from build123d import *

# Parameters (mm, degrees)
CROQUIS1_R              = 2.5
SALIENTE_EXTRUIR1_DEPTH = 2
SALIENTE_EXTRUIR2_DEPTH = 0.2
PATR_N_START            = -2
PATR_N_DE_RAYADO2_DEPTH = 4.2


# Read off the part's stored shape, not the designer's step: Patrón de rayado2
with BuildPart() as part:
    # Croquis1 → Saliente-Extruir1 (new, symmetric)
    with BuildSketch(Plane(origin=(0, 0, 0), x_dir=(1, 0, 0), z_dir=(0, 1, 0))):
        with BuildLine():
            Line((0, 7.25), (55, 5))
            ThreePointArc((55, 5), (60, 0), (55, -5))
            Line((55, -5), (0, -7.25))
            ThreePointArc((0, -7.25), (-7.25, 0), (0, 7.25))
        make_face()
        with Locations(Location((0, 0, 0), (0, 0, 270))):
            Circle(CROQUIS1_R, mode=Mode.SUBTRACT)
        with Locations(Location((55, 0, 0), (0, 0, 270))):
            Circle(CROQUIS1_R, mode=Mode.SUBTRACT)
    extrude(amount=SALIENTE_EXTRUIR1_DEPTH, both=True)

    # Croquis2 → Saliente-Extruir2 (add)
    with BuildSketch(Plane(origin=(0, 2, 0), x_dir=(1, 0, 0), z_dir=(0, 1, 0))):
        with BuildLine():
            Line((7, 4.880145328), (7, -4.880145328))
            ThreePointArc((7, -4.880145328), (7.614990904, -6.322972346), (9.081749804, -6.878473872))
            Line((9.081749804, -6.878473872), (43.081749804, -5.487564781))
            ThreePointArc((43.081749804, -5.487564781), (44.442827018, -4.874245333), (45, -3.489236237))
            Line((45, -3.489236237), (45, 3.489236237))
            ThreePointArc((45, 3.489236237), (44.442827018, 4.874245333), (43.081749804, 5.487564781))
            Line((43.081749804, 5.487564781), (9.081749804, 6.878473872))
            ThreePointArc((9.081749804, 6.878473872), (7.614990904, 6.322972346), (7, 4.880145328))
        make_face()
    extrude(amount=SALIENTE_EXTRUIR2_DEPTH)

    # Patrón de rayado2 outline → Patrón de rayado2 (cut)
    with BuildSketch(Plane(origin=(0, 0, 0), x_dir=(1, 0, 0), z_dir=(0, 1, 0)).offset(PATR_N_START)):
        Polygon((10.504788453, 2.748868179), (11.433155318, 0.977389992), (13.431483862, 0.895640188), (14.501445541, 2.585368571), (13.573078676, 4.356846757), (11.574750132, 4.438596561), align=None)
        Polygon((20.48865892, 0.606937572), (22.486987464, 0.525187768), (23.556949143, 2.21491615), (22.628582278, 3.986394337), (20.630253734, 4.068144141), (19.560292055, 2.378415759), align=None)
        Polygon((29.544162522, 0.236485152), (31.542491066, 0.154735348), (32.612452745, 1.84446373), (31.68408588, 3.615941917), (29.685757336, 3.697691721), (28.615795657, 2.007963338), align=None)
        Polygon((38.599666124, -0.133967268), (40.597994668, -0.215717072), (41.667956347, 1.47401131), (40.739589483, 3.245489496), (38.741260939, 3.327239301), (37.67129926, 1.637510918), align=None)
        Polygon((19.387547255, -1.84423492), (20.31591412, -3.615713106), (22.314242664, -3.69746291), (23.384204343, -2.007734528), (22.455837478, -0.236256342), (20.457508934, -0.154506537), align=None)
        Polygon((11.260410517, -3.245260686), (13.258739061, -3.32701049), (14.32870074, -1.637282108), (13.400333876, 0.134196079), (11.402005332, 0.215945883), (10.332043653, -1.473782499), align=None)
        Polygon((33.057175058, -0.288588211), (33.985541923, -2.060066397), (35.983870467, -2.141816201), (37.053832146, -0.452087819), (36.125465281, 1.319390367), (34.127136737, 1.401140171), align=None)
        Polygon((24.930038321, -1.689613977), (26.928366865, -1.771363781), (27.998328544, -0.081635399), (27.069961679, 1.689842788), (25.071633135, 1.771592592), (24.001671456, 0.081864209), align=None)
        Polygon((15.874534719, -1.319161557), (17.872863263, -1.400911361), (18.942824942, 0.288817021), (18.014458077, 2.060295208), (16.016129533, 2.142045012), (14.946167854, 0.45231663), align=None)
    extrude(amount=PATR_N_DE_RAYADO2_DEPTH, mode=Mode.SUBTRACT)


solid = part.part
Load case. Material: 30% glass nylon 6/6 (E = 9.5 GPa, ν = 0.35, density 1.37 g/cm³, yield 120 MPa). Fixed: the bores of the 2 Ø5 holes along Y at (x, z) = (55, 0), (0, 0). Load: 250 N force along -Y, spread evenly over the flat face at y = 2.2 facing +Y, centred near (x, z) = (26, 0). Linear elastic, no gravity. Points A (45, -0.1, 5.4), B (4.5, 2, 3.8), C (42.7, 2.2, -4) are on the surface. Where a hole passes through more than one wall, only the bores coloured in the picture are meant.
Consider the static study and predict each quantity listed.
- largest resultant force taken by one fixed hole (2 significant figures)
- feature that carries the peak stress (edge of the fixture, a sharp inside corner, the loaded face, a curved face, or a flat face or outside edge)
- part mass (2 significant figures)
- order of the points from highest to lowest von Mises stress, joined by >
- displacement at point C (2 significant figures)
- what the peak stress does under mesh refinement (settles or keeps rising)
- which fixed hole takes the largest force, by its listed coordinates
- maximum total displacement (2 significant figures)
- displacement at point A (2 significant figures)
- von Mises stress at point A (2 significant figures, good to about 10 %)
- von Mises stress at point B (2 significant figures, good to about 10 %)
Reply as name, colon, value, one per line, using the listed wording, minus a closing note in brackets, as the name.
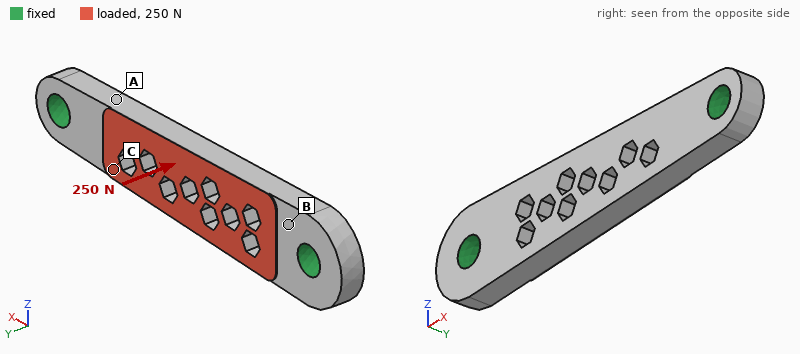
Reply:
largest resultant force taken by one fixed hole: 140 N
feature that carries the peak stress: edge of the fixture
part mass: 3.7 g
order of the points from highest to lowest von Mises stress, joined by >: B > A > C
displacement at point C: 0.10 mm
what the peak stress does under mesh refinement: keeps rising
which fixed hole takes the largest force, by its listed coordinates: (0, 0)
maximum total displacement: 0.23 mm
displacement at point A: 0.068 mm
von Mises stress at point A: 11 MPa
von Mises stress at point B: 25 MPa
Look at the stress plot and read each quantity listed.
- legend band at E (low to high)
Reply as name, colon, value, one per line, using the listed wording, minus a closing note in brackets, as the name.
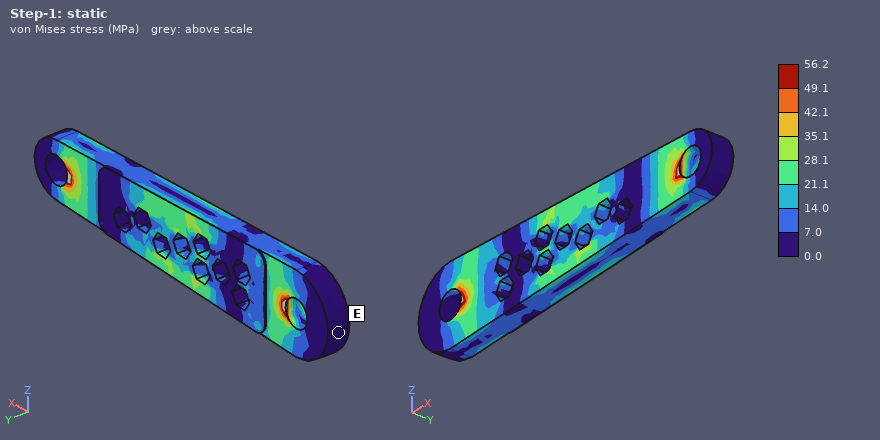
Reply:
legend band at E: 0.0 to 7.0 MPa
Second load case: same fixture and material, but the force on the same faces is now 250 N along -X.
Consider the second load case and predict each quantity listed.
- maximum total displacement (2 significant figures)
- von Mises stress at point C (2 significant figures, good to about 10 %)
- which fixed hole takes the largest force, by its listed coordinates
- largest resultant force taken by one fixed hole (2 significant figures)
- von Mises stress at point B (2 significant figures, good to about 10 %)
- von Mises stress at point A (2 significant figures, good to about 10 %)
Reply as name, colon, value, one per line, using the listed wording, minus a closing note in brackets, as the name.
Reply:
maximum total displacement: 8.2 µm
von Mises stress at point C: 3.9 MPa
which fixed hole takes the largest force, by its listed coordinates: (0, 0)
largest resultant force taken by one fixed hole: 130 N
von Mises stress at point B: 2.8 MPa
von Mises stress at point A: 2.8 MPa
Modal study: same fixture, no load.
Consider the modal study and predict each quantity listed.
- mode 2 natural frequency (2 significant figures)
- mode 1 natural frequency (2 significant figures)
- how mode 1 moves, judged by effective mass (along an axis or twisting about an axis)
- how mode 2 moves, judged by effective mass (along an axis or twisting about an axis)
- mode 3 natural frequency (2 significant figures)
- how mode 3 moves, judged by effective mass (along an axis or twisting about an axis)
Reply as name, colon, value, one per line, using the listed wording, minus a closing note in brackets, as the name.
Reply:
mode 2 natural frequency: 7500 Hz
mode 1 natural frequency: 4000 Hz
how mode 1 moves, judged by effective mass: along Y
how mode 2 moves, judged by effective mass: along Z
mode 3 natural frequency: 8200 Hz
how mode 3 moves, judged by effective mass: twisting about X
